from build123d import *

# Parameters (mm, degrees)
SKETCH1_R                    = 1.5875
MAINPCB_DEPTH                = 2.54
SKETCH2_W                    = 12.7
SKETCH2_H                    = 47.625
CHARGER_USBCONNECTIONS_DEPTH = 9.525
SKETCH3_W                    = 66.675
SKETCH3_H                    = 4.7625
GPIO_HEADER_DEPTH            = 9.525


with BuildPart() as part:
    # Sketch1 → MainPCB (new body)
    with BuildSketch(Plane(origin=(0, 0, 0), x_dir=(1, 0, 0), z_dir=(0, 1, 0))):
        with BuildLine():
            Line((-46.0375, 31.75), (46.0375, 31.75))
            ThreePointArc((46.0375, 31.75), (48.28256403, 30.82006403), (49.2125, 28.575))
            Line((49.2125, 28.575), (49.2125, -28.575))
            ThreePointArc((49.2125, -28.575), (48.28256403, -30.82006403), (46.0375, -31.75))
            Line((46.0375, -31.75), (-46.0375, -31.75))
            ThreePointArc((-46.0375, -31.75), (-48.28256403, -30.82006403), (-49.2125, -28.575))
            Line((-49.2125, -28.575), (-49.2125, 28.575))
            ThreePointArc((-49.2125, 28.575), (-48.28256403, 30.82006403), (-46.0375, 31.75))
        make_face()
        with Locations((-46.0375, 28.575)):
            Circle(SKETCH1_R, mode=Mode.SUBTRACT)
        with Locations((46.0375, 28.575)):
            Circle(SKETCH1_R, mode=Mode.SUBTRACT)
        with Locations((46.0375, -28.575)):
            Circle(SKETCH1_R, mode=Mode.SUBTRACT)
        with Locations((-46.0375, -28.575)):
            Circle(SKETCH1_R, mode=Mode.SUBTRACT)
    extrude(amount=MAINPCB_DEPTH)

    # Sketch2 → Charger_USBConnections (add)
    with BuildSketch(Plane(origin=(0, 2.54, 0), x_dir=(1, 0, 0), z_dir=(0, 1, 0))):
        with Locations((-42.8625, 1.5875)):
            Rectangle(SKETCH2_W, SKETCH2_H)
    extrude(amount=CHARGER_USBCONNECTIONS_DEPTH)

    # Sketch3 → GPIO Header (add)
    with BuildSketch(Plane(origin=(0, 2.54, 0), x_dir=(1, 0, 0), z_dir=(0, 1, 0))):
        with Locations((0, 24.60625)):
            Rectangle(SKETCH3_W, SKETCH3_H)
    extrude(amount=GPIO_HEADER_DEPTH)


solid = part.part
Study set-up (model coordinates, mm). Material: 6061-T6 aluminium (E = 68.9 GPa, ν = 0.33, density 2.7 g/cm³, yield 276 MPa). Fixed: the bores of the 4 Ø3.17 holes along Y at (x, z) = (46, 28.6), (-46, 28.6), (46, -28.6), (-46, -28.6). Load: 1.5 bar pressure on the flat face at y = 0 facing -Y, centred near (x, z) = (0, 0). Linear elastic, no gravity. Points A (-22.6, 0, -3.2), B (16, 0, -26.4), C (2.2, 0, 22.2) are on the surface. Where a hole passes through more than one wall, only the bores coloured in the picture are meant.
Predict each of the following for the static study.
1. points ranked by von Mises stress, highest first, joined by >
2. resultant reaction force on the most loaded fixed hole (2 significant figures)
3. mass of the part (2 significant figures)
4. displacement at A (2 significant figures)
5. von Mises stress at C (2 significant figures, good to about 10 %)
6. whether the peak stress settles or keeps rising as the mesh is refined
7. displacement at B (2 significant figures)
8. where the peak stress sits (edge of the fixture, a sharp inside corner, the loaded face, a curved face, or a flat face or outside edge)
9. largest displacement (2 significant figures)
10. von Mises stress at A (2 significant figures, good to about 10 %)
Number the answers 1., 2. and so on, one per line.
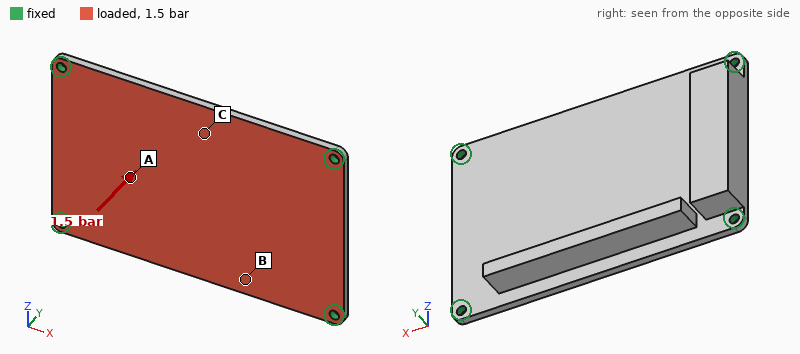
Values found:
1. C > A > B
2. 320 N
3. 66 g
4. 0.14 mm
5. 43 MPa
6. keeps rising
7. 0.067 mm
8. edge of the fixture
9. 0.34 mm
10. 28 MPa
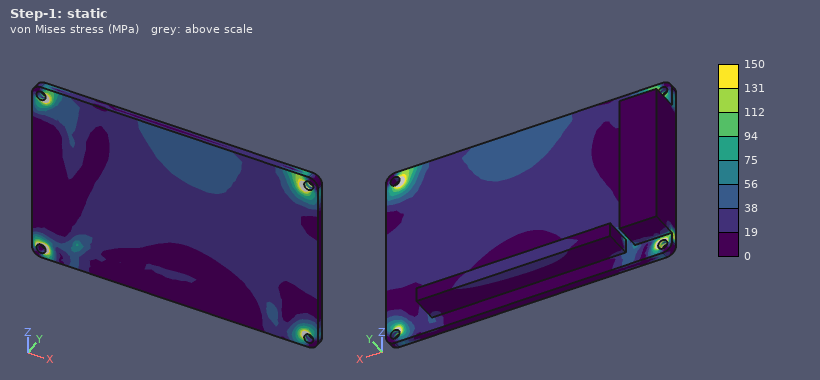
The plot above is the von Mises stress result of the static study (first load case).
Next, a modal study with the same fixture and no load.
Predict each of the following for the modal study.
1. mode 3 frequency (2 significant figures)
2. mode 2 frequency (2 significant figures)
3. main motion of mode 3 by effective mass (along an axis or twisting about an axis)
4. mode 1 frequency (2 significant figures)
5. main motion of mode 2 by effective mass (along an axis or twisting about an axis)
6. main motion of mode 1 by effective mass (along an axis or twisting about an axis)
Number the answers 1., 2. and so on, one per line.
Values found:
1. 3600 Hz
2. 3100 Hz
3. twisting about Z
4. 1600 Hz
5. along Y
6. along Y
